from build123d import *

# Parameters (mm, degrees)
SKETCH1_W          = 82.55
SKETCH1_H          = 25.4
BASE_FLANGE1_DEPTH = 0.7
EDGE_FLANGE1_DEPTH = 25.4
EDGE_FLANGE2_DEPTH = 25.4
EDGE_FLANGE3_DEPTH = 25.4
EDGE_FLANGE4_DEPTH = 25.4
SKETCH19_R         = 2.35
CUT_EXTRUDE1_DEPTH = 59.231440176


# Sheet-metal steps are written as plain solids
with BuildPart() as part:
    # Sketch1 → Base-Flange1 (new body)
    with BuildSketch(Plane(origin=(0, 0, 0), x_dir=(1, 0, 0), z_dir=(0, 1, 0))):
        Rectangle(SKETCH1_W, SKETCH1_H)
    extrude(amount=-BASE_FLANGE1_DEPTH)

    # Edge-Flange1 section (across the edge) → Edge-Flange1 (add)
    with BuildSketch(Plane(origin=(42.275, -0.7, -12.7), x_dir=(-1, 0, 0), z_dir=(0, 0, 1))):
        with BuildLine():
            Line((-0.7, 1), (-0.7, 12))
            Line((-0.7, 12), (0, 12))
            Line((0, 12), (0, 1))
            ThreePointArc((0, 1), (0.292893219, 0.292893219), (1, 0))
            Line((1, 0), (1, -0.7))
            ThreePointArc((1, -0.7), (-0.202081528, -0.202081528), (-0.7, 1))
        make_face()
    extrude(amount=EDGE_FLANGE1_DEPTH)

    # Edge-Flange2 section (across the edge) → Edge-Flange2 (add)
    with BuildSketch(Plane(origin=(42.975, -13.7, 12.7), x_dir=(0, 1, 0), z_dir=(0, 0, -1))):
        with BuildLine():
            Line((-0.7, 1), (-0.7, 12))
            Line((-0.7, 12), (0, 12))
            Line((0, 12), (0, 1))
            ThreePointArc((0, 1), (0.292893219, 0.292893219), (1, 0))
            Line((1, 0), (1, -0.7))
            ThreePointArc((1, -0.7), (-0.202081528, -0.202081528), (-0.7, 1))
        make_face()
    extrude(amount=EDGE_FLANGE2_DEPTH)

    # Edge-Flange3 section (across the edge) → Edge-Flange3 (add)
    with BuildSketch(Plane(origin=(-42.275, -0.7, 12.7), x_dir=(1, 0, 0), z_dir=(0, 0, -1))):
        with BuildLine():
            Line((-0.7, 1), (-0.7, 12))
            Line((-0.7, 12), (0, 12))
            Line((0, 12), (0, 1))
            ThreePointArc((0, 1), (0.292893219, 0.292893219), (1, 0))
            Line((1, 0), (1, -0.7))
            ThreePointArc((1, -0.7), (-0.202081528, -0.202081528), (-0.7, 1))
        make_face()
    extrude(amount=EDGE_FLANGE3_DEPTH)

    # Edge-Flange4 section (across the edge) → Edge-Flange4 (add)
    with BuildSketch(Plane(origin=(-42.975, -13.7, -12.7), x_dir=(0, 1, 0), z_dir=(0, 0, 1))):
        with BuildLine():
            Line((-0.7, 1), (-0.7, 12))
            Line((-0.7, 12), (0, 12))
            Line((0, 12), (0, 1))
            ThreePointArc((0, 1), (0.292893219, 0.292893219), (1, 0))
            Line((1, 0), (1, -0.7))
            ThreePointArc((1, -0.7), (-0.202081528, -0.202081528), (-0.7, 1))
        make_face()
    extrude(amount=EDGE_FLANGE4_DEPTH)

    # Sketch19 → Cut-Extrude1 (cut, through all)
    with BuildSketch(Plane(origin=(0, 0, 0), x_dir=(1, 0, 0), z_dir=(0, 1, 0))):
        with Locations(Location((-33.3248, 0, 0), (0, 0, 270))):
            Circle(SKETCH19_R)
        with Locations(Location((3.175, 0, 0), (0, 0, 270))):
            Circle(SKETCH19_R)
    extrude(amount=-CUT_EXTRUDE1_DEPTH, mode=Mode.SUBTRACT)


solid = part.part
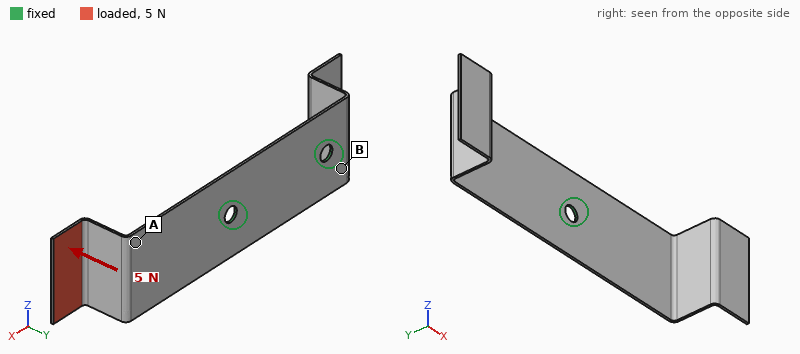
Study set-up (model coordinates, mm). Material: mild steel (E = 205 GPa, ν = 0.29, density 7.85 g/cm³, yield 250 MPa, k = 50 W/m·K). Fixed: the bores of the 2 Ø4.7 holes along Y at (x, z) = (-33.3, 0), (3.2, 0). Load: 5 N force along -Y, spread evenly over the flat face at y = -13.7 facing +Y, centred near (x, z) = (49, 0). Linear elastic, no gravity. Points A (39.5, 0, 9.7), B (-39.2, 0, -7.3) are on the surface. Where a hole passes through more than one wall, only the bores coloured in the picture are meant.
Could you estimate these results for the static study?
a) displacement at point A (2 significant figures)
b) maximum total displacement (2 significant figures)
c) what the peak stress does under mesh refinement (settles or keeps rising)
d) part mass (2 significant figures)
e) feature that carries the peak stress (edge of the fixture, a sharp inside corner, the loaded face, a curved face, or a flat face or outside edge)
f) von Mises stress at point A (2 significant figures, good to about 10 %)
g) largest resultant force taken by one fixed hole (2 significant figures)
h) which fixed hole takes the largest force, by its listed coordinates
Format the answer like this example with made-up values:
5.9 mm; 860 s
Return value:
0.69 mm; 1.3 mm; keeps rising; 19 g; edge of the fixture; 23 MPa; 5.5 N; (3.2, 0)
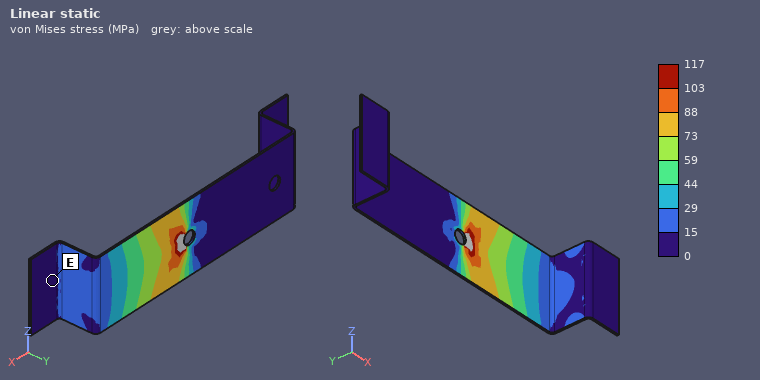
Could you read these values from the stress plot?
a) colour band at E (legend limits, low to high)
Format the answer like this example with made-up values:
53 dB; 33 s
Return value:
0 to 15 MPa
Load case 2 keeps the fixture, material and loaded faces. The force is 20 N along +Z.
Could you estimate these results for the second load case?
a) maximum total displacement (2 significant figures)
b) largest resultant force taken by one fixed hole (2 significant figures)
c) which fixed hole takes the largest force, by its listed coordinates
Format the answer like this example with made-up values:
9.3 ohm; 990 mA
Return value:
0.74 mm; 39 N; (3.2, 0)
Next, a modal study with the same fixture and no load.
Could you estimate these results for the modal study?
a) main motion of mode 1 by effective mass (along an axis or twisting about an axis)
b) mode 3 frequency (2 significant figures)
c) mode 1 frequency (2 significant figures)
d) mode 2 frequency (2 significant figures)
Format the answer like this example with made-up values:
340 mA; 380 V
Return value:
along Y; 690 Hz; 180 Hz; 490 Hz
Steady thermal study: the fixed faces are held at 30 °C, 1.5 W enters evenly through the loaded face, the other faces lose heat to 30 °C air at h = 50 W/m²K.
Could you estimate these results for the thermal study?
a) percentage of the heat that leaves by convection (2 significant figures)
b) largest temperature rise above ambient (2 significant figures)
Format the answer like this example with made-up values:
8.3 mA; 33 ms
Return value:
93 %; 29 K
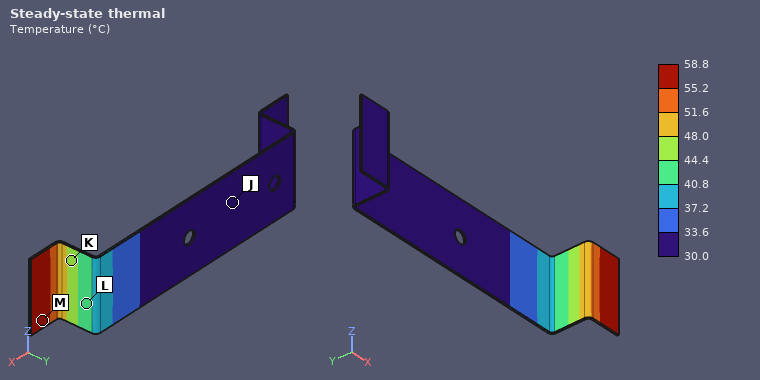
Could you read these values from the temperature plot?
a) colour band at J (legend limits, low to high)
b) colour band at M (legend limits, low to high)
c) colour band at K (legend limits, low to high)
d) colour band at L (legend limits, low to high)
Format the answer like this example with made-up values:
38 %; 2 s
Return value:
30.0 to 33.6 °C; 55.2 to 58.8 °C; 44.4 to 48.0 °C; 40.8 to 44.4 °C
